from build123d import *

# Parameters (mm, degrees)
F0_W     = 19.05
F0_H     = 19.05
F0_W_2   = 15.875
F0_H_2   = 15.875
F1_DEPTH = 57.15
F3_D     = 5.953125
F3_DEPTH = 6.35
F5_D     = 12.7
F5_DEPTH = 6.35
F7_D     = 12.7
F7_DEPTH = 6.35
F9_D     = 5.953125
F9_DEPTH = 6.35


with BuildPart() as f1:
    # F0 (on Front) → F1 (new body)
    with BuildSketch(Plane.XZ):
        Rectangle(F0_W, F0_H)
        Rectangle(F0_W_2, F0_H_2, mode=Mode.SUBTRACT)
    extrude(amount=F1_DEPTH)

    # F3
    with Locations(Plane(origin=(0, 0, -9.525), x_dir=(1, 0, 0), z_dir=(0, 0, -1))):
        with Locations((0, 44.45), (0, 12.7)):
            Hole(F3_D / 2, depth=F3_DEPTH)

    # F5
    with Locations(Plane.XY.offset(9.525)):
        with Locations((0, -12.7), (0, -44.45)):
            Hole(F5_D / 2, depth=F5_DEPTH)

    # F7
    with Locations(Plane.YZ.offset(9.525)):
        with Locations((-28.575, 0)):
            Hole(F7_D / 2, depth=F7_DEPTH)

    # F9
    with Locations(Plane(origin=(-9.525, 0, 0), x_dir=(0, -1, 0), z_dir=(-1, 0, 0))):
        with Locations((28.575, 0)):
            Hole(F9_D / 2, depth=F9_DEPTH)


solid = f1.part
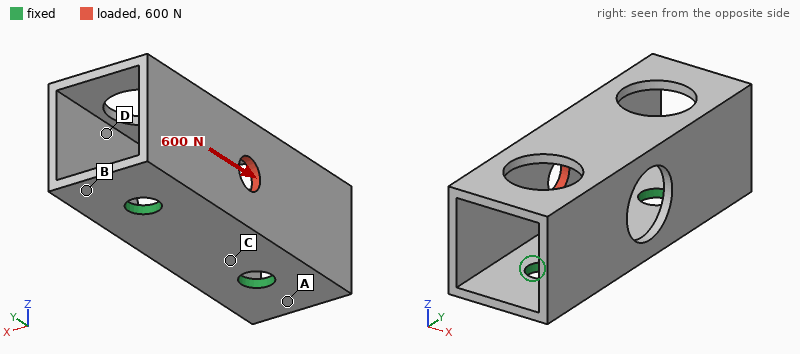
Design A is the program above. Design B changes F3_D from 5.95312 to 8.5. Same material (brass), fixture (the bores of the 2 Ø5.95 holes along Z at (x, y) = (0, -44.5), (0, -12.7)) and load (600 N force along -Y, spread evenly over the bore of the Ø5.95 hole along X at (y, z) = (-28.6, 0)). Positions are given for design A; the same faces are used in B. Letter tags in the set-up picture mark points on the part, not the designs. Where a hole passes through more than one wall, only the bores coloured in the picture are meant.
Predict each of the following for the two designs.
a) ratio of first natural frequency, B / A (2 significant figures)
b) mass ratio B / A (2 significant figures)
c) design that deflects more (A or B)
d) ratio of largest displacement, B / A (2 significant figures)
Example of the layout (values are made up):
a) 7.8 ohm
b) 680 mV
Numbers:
a) 1.2
b) 0.98
c) A
d) 0.70
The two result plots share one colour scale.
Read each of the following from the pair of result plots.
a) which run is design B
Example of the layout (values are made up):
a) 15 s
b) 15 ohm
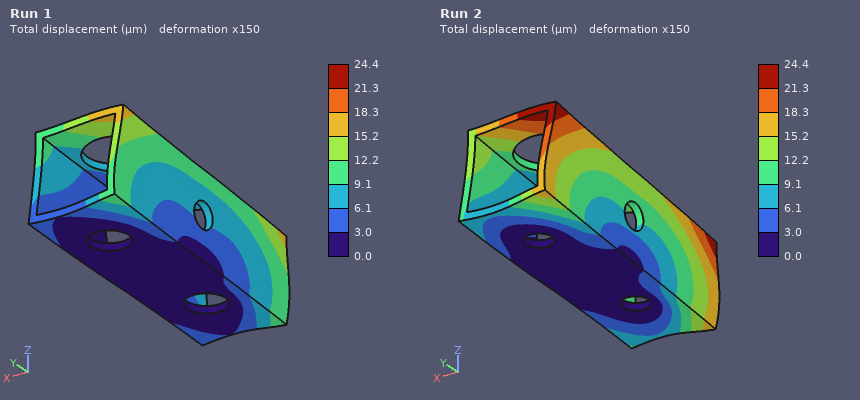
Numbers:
a) Run 1
